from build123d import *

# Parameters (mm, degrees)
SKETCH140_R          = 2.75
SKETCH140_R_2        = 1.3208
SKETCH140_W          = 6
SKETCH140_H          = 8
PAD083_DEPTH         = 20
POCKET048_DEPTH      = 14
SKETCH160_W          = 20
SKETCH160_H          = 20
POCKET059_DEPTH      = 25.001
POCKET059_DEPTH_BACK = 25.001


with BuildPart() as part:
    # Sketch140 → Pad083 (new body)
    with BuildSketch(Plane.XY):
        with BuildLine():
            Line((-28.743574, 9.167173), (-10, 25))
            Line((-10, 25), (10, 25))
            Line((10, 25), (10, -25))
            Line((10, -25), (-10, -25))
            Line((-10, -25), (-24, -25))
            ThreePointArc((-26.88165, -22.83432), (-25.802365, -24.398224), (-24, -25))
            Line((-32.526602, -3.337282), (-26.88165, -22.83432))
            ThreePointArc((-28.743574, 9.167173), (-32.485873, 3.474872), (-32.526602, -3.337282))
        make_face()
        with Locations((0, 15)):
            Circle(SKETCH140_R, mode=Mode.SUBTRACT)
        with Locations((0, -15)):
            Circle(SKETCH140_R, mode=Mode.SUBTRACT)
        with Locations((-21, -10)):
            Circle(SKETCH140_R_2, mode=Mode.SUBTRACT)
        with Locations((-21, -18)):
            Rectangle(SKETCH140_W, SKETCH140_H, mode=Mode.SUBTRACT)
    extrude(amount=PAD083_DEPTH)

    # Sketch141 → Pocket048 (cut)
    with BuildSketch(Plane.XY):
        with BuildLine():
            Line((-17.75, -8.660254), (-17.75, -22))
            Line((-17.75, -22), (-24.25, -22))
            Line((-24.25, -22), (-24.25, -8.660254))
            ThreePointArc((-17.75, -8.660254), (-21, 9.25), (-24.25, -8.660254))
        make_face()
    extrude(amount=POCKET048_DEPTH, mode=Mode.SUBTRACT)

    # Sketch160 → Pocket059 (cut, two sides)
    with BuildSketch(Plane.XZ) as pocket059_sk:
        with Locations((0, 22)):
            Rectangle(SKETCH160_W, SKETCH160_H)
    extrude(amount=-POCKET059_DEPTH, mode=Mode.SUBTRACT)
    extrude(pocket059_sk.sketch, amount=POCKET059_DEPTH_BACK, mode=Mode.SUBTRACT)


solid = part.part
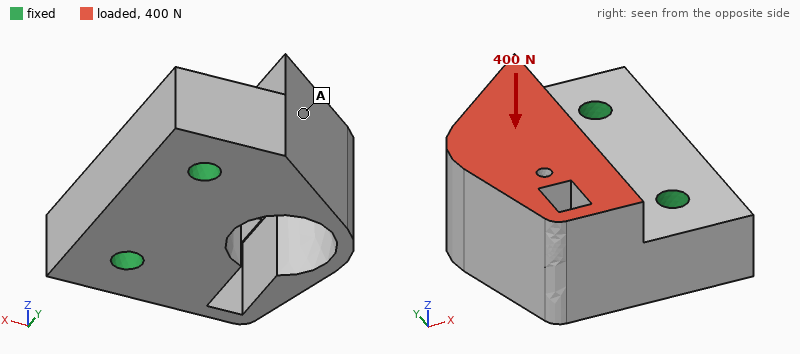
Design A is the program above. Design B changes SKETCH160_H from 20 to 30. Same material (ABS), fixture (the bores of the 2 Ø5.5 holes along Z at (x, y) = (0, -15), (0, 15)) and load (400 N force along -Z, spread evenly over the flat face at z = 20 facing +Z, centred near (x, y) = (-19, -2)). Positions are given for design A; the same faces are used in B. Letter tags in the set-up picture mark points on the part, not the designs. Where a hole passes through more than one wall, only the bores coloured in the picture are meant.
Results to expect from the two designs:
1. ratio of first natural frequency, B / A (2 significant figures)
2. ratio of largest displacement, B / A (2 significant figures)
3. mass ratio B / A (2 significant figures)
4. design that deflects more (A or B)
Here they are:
0.52
3.3
0.79
B
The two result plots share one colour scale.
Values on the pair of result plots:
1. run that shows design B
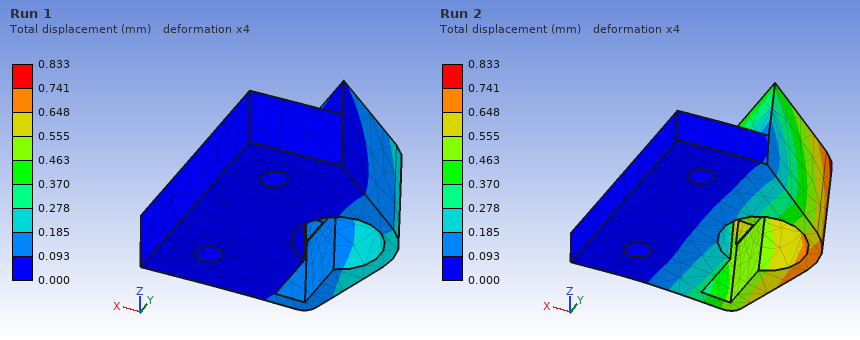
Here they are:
Run 2
